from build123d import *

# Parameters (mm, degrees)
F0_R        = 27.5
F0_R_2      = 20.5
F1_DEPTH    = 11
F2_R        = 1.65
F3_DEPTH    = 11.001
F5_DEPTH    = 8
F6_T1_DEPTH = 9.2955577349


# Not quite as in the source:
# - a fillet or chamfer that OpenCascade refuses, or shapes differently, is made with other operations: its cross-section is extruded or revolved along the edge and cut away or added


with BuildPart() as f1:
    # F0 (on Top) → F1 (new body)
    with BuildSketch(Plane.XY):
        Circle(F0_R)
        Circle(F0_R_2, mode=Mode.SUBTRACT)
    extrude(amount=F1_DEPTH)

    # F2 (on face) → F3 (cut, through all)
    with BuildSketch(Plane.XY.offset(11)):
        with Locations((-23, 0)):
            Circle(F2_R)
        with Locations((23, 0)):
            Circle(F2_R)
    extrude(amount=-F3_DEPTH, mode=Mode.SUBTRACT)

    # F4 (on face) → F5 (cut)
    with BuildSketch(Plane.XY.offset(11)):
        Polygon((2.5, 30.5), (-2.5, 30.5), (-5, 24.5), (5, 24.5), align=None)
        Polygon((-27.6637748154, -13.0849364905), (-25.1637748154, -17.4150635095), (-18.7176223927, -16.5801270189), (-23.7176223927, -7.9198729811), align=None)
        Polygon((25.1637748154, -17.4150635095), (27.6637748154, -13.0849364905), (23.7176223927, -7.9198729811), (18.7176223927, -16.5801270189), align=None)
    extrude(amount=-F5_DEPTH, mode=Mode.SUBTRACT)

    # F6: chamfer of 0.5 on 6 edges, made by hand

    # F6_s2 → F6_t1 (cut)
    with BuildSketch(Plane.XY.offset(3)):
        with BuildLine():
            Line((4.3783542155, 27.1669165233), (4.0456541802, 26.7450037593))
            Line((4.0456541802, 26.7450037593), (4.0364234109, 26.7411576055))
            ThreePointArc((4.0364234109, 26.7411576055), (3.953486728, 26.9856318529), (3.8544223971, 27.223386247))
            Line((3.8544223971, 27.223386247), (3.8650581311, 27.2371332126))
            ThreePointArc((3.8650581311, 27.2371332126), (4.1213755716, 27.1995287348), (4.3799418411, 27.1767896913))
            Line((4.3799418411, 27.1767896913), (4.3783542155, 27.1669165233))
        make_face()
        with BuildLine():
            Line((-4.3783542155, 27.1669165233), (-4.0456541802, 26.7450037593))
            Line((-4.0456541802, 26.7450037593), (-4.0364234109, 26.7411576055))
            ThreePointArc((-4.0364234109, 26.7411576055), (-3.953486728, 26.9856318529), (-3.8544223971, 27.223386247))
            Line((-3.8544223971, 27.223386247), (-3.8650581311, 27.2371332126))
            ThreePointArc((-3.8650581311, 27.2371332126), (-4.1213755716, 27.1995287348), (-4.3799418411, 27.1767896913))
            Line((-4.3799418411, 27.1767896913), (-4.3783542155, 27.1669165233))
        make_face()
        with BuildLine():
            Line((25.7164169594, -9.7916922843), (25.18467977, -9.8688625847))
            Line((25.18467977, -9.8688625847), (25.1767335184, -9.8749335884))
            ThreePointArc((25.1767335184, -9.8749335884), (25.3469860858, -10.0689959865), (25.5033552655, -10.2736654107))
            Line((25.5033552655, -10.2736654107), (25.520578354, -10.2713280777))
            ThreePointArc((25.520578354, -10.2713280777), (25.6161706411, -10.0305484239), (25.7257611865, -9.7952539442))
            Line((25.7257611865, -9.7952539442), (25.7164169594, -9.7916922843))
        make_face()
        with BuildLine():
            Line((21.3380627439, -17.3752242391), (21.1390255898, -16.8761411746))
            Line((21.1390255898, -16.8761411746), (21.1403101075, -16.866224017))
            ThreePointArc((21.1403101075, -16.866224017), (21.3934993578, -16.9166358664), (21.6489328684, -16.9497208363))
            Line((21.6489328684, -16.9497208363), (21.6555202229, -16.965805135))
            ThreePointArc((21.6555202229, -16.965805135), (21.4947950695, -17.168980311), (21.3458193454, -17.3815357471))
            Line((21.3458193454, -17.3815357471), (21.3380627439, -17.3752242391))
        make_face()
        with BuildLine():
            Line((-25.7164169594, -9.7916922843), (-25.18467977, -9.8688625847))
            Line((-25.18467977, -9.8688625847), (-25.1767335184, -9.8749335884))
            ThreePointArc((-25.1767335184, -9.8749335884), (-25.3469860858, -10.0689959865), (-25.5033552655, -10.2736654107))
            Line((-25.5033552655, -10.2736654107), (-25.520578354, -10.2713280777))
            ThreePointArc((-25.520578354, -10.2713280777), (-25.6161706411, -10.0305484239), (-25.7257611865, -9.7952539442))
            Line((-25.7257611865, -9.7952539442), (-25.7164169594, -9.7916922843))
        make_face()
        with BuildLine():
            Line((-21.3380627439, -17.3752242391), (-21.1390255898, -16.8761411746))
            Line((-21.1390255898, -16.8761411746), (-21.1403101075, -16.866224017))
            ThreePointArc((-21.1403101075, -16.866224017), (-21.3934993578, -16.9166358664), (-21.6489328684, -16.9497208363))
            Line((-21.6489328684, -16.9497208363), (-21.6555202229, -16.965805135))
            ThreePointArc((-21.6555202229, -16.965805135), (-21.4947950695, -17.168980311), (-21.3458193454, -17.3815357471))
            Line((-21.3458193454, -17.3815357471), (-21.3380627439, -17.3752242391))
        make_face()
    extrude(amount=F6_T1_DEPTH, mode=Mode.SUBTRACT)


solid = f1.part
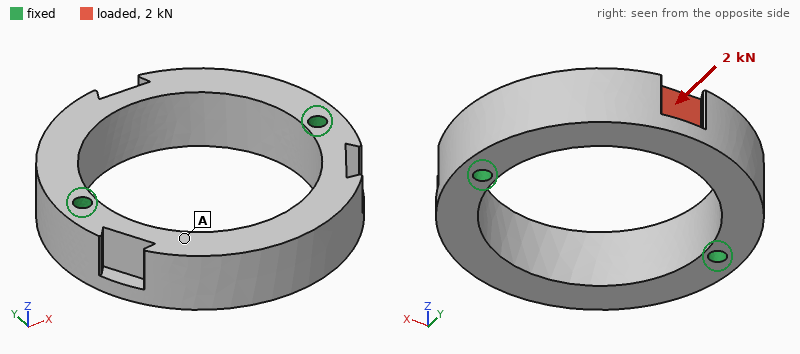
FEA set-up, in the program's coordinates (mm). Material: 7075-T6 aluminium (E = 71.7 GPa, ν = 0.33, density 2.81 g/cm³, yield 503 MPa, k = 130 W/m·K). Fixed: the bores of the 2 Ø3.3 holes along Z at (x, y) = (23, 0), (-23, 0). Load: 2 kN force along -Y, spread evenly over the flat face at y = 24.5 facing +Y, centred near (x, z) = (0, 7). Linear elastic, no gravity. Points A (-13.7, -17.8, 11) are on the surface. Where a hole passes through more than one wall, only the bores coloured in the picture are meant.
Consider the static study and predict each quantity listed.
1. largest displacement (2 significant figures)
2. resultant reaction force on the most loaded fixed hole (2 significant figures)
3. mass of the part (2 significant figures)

55 µm
1.4 kN
30 g
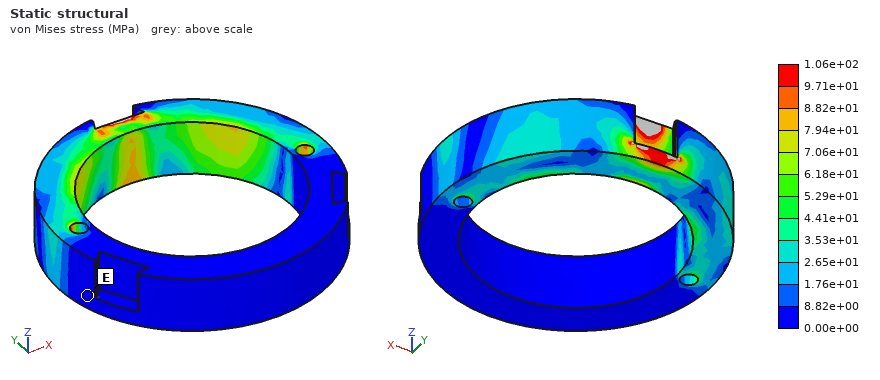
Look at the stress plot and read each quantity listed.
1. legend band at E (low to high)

0.00e+00 to 8.82e+00 MPa
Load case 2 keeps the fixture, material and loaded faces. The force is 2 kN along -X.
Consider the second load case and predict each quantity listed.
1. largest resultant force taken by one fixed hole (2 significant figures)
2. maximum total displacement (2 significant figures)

1.2 kN
44 µm
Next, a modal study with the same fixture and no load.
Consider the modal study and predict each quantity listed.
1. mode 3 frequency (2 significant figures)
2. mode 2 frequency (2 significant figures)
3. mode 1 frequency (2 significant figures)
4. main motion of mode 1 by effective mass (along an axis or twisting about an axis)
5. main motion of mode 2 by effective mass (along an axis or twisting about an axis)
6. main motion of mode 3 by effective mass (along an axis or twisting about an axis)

9900 Hz
7700 Hz
6800 Hz
along Z
along Z
twisting about Z
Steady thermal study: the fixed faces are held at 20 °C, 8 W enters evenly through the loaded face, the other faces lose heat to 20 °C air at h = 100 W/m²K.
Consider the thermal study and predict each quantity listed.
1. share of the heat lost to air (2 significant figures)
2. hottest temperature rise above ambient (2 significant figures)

20 %
14 K
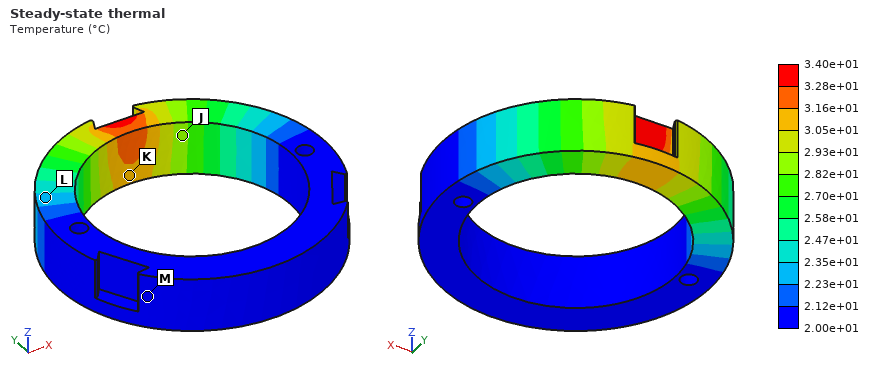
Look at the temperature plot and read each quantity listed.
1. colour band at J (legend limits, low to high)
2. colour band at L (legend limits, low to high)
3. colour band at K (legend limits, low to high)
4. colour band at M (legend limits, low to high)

2.82e+01 to 2.93e+01 °C
2.23e+01 to 2.35e+01 °C
3.05e+01 to 3.16e+01 °C
2.00e+01 to 2.12e+01 °C
